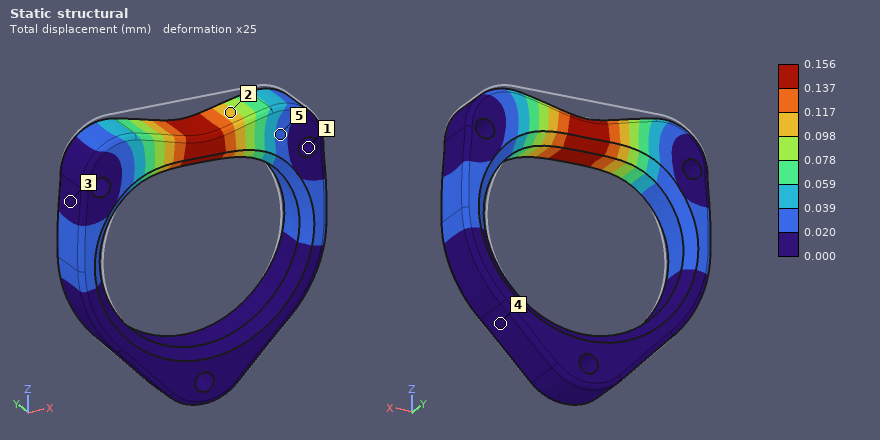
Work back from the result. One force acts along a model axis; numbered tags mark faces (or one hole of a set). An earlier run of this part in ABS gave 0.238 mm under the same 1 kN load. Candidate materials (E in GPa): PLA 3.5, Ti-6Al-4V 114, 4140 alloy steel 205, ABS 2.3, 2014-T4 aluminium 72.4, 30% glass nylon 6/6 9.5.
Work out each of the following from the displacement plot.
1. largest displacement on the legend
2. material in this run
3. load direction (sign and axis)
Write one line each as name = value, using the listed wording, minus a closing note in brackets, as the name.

largest displacement on the legend = 0.156 mm
material in this run = PLA
load direction = -Z
